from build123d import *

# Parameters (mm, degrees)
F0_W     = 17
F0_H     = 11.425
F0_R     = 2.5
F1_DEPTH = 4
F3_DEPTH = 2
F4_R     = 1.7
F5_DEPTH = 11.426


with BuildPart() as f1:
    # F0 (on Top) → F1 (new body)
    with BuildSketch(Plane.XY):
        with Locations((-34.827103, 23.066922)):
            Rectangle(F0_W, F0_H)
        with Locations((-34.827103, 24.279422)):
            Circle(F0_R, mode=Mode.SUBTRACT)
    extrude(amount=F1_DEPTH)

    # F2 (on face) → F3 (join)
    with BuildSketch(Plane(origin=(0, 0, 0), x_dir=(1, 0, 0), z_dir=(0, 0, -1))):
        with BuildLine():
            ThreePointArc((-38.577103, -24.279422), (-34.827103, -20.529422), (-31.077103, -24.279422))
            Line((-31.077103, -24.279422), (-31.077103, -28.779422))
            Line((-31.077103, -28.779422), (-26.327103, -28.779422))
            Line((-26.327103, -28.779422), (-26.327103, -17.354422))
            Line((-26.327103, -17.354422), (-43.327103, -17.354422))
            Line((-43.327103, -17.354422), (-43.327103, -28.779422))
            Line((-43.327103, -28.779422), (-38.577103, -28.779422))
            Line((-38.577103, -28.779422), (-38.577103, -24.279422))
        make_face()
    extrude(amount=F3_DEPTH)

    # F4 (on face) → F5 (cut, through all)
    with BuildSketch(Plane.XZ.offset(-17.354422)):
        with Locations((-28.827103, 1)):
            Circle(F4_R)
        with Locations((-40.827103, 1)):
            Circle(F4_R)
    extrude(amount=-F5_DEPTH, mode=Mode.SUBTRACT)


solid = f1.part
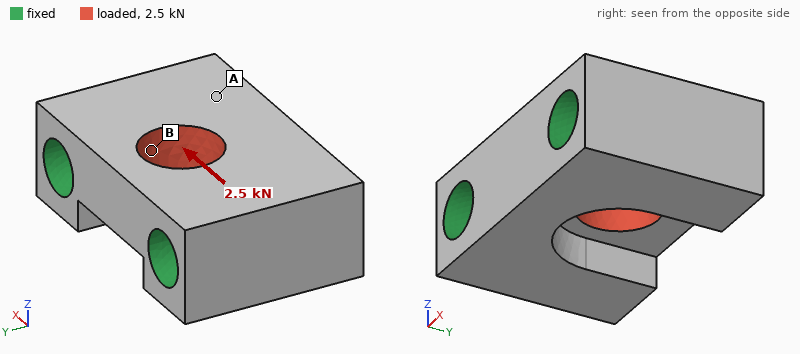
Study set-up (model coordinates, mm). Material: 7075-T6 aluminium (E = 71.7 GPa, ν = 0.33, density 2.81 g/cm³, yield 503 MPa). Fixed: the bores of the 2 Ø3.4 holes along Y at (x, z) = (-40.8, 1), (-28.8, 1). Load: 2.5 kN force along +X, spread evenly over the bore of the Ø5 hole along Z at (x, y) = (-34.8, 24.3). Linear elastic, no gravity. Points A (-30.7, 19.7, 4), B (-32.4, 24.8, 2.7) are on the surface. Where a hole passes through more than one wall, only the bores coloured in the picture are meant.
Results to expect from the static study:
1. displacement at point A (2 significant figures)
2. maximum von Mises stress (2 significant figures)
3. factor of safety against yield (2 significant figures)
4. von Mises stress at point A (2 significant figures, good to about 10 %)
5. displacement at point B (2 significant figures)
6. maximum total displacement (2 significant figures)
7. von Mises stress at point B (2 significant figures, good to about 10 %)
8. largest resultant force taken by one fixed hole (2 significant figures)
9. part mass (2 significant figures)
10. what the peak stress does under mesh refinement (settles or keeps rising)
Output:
0.52 µm
70 MPa
7.2
15 MPa
1.7 µm
2.5 µm
40 MPa
1.3 kN
2.2 g
settles
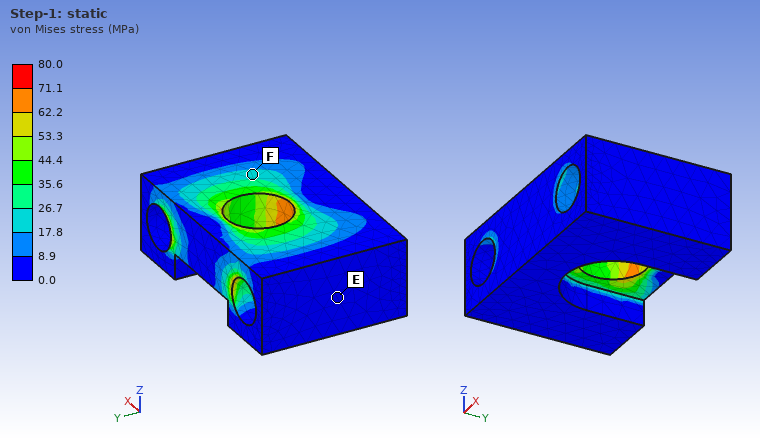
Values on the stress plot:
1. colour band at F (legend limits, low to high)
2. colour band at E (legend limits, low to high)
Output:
17.8 to 26.7 MPa
0.0 to 8.9 MPa
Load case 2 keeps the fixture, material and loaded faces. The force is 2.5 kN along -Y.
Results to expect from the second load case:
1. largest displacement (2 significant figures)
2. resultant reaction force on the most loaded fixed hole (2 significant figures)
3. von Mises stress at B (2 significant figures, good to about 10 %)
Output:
7.5 µm
1.3 kN
89 MPa
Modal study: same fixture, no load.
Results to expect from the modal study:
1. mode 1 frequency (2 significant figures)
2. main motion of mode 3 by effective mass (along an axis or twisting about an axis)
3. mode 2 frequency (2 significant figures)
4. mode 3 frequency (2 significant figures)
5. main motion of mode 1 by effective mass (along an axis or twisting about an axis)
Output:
140 kHz
along Y
140 kHz
160 kHz
along Z
